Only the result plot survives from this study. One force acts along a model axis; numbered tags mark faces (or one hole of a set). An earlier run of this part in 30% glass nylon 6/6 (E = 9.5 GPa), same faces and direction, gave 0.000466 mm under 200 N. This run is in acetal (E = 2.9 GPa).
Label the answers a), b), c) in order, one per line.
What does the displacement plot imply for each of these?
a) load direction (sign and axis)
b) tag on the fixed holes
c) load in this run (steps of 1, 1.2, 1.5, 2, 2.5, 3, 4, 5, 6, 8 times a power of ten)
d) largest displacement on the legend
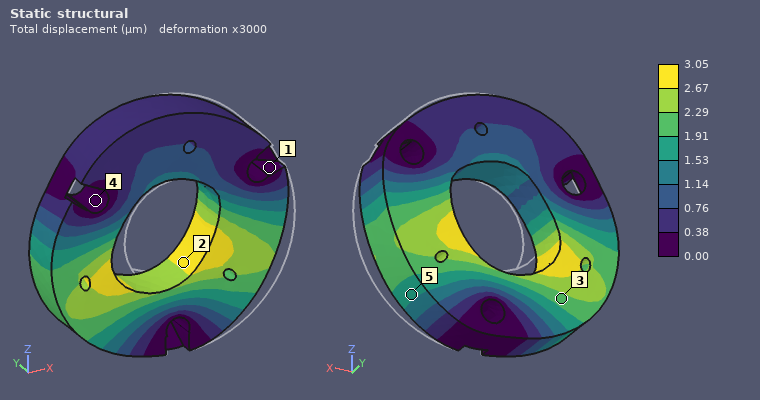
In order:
a) -X
b) 4
c) 400 N
d) 3.05 µm
